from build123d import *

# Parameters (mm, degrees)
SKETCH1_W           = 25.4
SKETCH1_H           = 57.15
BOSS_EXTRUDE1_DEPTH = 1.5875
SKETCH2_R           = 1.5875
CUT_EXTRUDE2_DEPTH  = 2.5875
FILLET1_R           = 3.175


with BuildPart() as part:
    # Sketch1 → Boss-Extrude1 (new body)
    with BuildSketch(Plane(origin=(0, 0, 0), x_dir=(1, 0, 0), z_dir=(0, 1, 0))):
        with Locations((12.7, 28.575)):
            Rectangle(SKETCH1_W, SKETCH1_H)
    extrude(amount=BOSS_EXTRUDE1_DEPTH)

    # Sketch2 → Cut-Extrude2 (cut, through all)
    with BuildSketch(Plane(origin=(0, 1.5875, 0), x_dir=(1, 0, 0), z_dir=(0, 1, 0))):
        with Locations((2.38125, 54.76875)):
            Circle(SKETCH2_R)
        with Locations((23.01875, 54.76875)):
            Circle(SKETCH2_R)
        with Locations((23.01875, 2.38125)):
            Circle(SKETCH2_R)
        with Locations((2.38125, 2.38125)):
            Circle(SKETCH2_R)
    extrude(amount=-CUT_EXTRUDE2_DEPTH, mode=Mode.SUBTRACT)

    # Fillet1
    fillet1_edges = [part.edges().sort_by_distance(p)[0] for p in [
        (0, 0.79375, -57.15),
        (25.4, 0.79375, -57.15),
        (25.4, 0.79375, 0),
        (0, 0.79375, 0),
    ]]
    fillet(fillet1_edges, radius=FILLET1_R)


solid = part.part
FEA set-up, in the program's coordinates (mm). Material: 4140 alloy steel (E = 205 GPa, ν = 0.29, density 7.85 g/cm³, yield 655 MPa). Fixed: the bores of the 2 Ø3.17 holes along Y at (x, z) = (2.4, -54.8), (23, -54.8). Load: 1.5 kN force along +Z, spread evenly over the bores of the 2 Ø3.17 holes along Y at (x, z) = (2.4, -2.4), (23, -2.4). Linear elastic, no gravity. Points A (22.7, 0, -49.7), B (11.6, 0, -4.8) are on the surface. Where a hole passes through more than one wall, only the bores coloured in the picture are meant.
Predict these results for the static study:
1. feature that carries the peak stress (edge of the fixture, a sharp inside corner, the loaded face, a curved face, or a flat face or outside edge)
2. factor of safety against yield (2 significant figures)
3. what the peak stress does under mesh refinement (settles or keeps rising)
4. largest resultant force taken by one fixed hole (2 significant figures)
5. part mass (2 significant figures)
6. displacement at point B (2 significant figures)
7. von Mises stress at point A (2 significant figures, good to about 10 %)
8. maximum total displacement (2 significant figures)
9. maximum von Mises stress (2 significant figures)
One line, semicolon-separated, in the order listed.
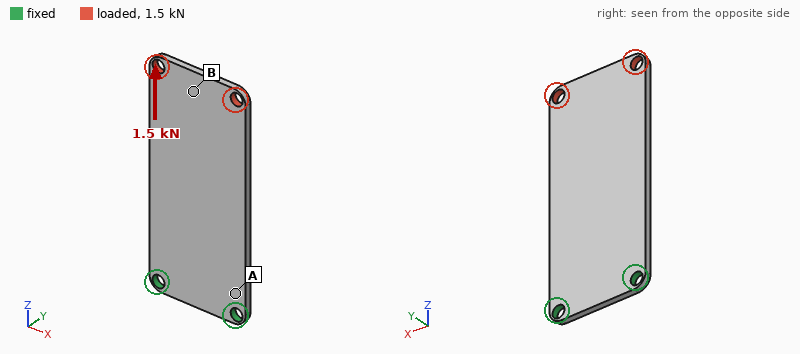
the loaded face; 1.5; settles; 770 N; 18 g; 8.6 µm; 64 MPa; 19 µm; 450 MPa
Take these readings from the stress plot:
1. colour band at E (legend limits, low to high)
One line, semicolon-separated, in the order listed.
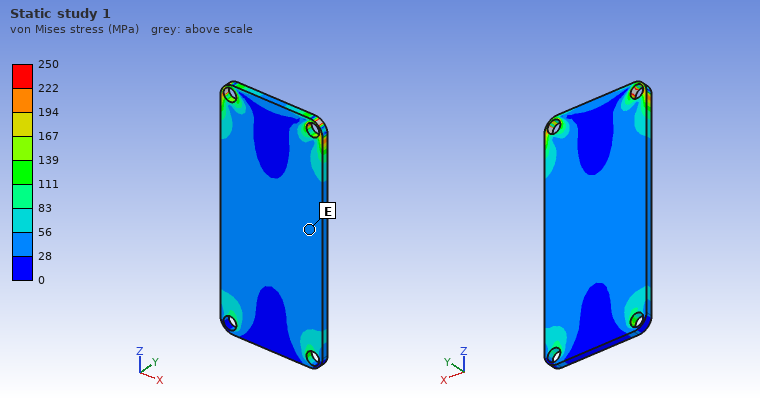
28 to 56 MPa
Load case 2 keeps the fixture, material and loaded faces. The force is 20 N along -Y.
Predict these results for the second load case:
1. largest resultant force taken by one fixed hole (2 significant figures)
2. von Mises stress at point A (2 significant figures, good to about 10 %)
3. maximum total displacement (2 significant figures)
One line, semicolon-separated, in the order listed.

10 N; 99 MPa; 0.60 mm
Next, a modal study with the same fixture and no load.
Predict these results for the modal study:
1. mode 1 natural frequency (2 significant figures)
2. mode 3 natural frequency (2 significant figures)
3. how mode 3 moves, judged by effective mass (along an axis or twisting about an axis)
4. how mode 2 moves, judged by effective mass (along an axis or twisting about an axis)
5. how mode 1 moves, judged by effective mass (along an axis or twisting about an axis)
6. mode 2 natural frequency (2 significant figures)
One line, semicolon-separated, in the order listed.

440 Hz; 2800 Hz; along Y; twisting about Z; along Y; 2100 Hz
